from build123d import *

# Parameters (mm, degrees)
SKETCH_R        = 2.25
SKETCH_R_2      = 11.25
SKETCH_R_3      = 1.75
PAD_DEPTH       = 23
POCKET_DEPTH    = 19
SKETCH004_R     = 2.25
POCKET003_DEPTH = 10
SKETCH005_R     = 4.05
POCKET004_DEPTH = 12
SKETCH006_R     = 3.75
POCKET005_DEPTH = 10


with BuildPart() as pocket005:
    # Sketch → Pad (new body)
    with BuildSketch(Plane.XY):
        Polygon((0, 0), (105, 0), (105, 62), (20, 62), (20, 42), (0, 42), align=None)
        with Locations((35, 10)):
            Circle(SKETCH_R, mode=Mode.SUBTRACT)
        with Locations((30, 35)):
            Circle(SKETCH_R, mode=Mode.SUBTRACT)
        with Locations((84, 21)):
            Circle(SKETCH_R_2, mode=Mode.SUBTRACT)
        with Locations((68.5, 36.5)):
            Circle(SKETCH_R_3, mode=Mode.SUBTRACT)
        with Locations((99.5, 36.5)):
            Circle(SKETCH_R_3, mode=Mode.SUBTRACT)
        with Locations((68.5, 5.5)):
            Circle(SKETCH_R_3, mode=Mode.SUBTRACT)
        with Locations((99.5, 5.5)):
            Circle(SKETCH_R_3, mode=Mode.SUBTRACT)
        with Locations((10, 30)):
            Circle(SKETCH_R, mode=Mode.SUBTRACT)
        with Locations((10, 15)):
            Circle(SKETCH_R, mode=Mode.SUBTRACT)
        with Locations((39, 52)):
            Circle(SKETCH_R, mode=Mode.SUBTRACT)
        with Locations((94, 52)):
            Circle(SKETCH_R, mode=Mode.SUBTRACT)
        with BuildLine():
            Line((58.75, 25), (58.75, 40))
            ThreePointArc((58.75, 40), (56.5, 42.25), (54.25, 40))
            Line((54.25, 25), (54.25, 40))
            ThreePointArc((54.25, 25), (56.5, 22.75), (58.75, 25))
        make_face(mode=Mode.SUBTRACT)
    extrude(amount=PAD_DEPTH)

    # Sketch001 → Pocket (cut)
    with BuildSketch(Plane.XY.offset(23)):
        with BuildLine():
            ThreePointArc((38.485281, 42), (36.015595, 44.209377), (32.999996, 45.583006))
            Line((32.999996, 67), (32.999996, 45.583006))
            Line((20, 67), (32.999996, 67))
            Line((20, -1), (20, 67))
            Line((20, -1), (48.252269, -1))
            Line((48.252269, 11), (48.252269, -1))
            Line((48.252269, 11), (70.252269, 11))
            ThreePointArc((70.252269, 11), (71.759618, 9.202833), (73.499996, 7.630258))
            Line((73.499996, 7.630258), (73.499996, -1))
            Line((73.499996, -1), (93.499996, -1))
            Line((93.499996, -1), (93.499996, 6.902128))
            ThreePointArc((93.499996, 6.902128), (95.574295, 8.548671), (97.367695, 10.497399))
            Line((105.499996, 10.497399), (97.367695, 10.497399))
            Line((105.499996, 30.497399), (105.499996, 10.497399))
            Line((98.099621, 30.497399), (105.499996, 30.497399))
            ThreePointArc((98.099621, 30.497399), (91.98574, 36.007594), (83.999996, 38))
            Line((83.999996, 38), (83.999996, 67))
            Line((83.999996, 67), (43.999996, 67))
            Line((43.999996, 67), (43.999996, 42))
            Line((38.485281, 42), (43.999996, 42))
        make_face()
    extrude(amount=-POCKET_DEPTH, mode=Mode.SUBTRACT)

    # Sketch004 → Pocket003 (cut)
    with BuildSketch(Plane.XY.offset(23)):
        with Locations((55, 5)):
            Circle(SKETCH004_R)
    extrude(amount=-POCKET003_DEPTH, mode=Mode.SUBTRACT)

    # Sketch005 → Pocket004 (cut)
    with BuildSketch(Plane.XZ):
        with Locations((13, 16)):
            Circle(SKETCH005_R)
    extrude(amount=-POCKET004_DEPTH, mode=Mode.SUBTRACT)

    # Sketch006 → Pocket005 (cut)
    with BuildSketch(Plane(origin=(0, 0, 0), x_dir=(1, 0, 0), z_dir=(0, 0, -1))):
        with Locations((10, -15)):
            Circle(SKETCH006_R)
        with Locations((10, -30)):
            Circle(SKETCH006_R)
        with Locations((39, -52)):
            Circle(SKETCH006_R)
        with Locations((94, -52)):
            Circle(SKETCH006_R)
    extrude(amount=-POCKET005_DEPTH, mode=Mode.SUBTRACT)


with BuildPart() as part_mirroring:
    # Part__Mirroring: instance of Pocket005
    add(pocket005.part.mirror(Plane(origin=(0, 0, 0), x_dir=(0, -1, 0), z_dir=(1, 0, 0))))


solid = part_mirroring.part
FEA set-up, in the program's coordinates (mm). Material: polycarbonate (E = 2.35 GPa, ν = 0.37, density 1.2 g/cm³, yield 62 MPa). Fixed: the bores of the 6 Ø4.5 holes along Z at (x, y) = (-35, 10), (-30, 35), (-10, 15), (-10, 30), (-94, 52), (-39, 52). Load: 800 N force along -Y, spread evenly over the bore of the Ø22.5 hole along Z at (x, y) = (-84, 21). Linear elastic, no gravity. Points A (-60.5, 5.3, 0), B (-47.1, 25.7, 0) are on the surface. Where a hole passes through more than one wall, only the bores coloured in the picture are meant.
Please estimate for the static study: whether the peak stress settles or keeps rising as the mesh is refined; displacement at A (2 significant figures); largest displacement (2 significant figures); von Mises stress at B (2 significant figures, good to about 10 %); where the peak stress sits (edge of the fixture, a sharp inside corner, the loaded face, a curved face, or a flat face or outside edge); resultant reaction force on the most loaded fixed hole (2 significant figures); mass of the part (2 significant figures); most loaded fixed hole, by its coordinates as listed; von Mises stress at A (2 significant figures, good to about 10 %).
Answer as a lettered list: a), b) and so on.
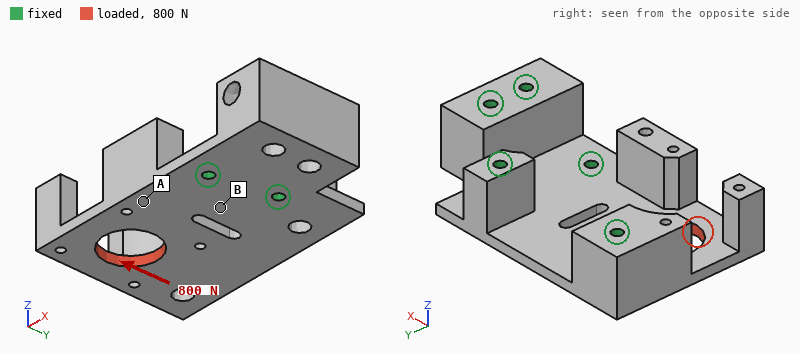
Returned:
a) keeps rising
b) 0.12 mm
c) 0.31 mm
d) 4.5 MPa
e) edge of the fixture
f) 530 N
g) 68 g
h) (-94, 52)
i) 1.6 MPa
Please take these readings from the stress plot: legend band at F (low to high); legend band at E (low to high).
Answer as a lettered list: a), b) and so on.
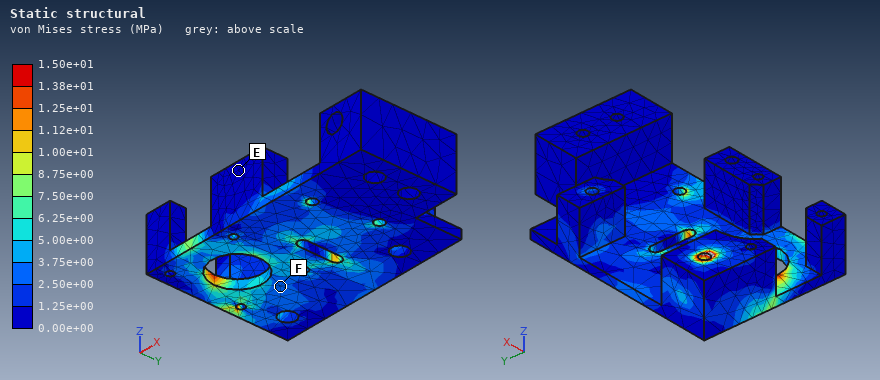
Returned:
a) 2.50e+00 to 3.75e+00 MPa
b) 0.00e+00 to 1.25e+00 MPa
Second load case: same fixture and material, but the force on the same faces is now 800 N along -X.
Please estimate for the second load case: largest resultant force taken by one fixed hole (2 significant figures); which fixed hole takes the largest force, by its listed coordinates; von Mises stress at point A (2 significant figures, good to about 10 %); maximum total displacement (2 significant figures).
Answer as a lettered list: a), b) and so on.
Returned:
a) 330 N
b) (-35, 10)
c) 3.9 MPa
d) 0.17 mm
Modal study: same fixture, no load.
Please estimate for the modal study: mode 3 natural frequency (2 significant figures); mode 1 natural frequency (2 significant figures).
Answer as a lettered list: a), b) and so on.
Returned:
a) 1200 Hz
b) 430 Hz
